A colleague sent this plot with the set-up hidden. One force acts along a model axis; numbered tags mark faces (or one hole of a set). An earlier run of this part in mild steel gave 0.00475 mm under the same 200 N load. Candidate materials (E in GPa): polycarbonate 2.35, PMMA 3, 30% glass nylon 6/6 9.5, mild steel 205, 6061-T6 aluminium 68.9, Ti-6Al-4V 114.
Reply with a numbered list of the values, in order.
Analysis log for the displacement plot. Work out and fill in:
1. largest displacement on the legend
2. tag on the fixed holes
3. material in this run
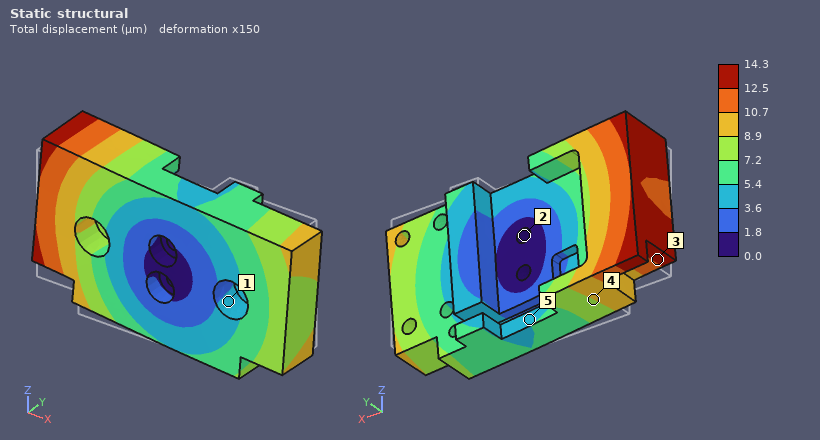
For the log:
1. 14.3 µm
2. 2
3. 6061-T6 aluminium
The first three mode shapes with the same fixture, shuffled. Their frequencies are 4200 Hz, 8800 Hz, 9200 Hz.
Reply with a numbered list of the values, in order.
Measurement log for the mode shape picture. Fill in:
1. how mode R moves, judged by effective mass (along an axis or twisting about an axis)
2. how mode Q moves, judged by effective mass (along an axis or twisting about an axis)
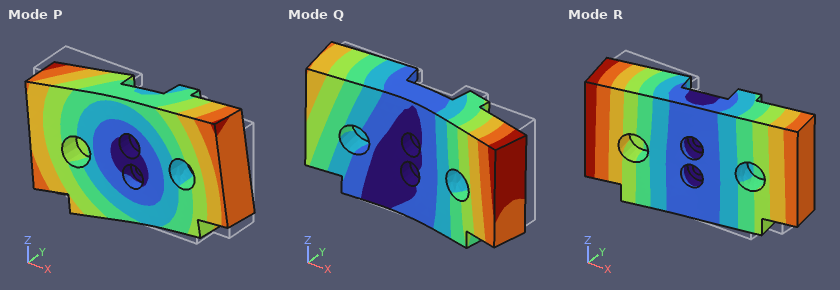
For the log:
1. twisting about Z
2. along Y
